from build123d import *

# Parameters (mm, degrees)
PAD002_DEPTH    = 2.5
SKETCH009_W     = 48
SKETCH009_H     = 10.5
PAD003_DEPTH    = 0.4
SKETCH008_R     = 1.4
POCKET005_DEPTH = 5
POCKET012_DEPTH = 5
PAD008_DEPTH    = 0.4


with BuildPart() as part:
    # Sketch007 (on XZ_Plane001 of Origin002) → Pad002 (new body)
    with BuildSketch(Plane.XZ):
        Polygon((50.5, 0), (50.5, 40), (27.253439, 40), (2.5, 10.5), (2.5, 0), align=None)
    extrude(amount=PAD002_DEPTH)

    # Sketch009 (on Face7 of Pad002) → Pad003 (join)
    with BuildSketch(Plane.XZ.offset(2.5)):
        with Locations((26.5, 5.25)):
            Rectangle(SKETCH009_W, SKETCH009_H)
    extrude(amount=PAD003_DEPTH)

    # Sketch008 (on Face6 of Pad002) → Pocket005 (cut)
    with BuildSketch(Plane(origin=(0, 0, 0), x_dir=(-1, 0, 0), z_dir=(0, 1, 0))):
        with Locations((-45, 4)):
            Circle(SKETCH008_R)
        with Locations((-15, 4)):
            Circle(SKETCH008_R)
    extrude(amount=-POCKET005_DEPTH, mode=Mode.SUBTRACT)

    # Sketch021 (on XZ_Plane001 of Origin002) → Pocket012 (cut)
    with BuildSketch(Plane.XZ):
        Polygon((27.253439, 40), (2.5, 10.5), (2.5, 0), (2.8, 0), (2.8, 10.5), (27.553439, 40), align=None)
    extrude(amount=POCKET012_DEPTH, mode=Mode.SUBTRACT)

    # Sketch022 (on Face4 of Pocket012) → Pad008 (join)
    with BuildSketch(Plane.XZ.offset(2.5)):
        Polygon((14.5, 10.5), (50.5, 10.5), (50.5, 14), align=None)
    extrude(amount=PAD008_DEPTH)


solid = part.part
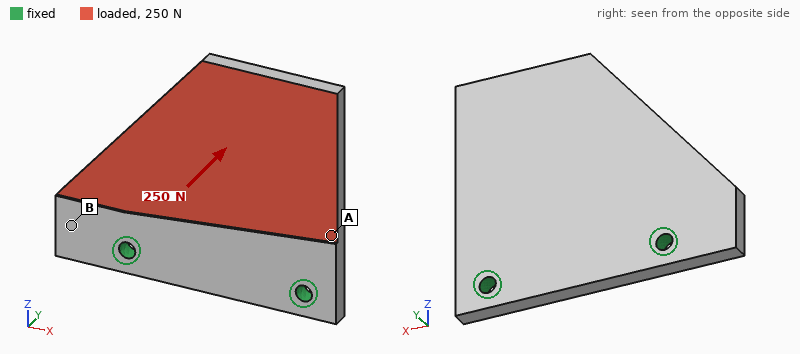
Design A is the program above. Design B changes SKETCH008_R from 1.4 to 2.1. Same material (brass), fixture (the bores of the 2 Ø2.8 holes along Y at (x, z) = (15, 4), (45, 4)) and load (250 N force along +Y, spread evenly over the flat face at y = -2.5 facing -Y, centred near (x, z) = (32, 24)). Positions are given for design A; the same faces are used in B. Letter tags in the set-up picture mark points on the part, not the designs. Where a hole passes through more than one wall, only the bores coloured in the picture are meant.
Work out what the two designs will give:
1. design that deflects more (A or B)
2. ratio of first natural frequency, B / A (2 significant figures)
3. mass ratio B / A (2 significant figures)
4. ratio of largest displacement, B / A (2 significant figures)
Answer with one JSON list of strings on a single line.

["A", "1.1", "0.99", "0.89"]
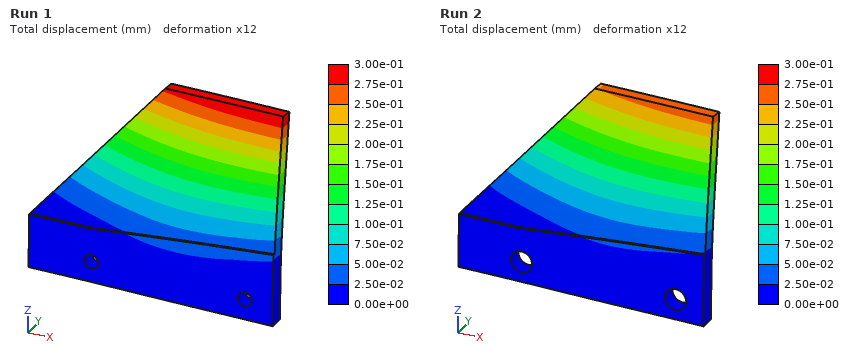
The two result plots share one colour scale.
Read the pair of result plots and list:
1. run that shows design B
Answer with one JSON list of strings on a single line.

["Run 2"]
